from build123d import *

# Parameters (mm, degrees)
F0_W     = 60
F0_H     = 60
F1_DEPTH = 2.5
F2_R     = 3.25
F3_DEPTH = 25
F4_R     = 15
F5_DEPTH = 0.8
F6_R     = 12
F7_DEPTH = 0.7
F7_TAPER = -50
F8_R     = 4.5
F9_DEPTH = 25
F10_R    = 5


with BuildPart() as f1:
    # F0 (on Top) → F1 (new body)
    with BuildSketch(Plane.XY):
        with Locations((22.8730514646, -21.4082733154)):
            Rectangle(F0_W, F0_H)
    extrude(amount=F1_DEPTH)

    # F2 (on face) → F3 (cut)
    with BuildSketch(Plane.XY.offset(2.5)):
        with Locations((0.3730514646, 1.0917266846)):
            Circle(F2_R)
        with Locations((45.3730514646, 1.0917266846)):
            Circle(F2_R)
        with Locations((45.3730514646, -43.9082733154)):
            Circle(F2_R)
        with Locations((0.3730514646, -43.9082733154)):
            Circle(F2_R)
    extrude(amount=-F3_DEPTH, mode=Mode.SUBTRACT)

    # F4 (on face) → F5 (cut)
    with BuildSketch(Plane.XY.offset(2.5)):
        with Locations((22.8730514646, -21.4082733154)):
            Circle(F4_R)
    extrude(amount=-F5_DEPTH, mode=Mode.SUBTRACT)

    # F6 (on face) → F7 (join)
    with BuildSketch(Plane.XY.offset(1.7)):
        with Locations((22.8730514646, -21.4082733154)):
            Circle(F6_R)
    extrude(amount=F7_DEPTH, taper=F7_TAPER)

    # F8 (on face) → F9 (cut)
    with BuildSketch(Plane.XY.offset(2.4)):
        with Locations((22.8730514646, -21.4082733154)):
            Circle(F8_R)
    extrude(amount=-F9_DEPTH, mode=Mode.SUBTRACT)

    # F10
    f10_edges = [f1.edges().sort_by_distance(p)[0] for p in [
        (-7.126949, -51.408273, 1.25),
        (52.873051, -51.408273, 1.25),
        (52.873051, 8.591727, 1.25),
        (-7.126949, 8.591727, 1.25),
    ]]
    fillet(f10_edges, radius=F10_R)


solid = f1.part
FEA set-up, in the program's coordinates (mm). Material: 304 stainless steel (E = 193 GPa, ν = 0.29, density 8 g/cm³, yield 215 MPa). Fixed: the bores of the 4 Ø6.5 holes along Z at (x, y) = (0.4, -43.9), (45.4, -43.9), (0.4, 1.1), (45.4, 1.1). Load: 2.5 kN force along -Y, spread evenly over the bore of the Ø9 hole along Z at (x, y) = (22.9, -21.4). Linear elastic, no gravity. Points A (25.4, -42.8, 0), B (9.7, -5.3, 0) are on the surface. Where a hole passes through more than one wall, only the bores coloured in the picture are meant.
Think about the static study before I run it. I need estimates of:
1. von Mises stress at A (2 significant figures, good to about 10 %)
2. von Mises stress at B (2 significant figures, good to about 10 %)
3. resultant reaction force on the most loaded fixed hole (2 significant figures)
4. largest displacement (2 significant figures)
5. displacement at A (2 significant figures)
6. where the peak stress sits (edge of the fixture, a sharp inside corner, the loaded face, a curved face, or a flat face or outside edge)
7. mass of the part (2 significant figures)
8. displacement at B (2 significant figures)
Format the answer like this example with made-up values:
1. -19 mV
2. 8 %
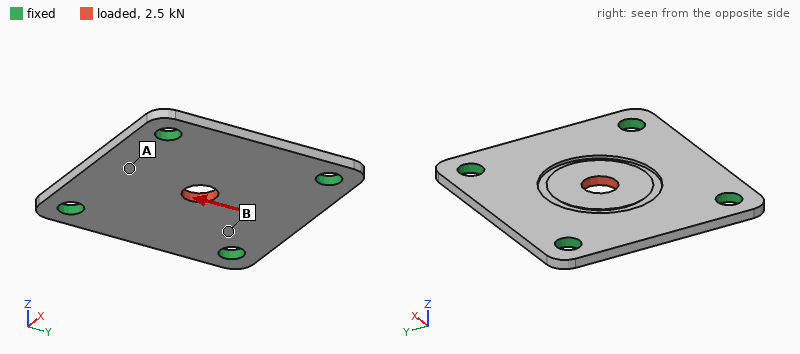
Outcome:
1. 9.4 MPa
2. 22 MPa
3. 690 N
4. 4.3 µm
5. 2.5 µm
6. the loaded face
7. 66 g
8. 1.5 µm
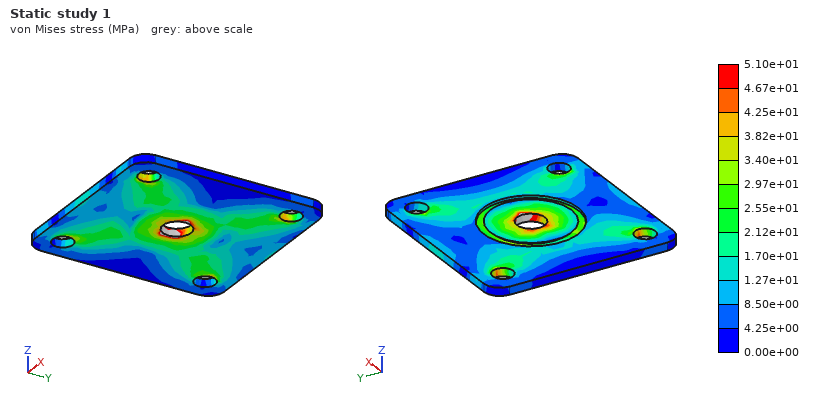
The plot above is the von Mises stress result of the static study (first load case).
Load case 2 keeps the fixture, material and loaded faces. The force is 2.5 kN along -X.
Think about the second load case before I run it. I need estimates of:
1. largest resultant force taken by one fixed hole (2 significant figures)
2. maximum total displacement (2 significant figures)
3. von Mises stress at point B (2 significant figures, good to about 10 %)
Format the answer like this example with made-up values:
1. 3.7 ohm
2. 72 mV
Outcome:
1. 690 N
2. 4.3 µm
3. 20 MPa
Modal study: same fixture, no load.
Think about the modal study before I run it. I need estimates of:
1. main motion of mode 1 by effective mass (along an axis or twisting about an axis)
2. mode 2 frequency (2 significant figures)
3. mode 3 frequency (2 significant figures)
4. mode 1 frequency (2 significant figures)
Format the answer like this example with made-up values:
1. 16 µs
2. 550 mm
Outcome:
1. along Z
2. 7800 Hz
3. 7800 Hz
4. 5100 Hz
